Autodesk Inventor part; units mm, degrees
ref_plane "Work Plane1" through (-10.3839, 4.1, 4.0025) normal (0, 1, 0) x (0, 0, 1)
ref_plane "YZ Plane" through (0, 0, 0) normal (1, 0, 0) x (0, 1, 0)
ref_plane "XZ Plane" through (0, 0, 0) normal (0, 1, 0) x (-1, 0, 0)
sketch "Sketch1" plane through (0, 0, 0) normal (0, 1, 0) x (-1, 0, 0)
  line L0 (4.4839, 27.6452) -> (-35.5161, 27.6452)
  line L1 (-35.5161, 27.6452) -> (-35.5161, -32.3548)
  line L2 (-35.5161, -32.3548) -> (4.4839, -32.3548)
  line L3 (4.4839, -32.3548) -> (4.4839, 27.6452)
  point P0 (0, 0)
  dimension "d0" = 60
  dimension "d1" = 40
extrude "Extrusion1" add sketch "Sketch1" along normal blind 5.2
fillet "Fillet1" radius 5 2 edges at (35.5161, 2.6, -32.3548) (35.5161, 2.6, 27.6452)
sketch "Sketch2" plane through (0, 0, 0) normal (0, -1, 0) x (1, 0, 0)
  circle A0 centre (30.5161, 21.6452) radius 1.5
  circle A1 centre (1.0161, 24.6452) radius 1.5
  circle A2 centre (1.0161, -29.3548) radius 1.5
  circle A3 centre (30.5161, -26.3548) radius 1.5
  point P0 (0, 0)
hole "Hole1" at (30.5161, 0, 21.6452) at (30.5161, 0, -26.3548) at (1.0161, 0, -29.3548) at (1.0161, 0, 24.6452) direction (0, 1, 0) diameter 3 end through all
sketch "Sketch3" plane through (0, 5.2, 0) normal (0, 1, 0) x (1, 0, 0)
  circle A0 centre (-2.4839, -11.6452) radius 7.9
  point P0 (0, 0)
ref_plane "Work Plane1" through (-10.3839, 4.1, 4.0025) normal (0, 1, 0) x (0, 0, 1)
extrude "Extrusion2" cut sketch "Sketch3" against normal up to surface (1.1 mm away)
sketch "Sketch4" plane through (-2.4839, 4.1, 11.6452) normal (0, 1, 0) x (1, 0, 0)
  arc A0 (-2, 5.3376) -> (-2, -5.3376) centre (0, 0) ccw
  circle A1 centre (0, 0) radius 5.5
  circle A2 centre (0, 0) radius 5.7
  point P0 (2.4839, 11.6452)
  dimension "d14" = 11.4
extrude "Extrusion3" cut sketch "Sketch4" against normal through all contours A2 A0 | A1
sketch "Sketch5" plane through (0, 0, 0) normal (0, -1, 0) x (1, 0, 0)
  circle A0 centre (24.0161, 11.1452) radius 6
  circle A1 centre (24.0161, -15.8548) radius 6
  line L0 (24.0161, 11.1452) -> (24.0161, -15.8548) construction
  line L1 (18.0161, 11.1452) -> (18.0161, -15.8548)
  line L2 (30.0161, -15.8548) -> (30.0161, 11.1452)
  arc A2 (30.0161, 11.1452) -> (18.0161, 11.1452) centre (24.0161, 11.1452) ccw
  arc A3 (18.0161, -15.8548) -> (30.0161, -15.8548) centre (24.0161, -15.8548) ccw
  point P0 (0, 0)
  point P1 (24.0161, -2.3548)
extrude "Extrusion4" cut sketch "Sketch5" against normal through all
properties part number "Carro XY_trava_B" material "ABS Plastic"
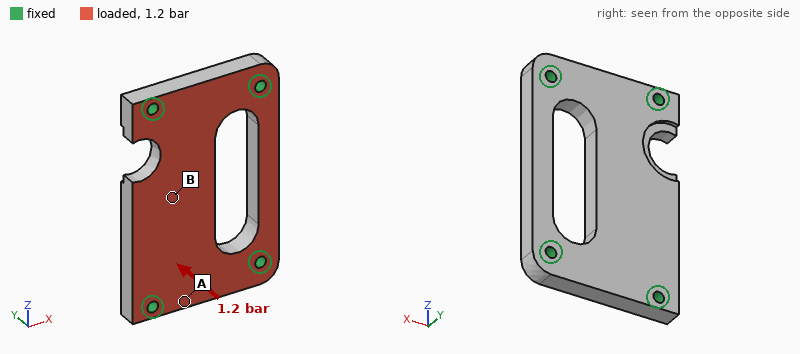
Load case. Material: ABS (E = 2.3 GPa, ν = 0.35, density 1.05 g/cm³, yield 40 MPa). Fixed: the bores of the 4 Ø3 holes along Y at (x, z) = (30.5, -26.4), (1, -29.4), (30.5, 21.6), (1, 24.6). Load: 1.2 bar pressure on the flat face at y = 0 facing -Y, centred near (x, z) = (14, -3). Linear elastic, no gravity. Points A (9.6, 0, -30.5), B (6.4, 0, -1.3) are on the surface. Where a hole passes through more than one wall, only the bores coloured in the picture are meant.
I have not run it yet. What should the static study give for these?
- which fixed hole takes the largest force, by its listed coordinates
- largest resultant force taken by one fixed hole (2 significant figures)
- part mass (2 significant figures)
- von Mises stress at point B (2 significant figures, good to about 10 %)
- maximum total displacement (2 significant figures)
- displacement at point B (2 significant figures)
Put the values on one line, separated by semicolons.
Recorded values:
(1, -29.4); 66 N; 10 g; 3.5 MPa; 0.16 mm; 0.14 mm
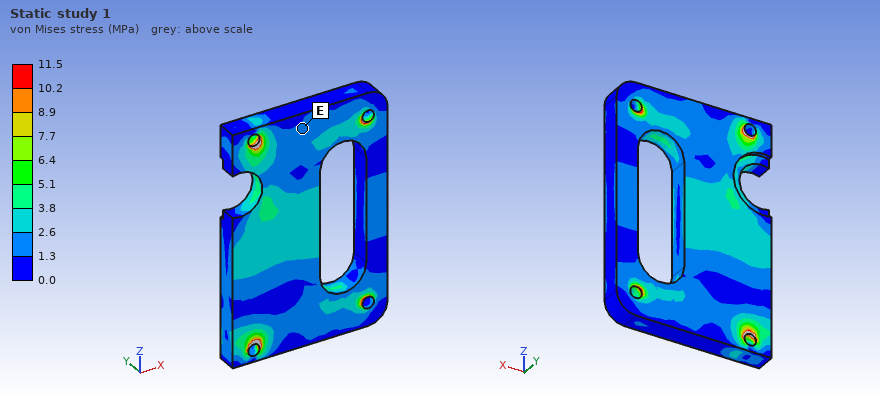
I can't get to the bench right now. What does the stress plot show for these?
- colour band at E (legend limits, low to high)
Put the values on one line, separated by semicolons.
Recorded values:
1.3 to 2.6 MPa
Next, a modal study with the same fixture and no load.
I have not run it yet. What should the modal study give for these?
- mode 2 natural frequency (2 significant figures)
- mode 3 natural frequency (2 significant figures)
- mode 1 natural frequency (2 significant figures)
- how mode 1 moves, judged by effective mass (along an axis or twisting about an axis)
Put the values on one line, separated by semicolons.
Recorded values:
3700 Hz; 4100 Hz; 2200 Hz; along Y
